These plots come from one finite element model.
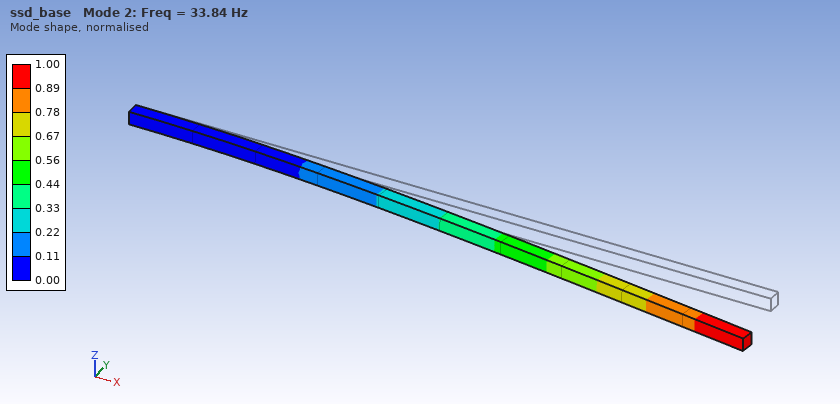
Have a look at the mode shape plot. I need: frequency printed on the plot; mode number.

33.84 Hz
2
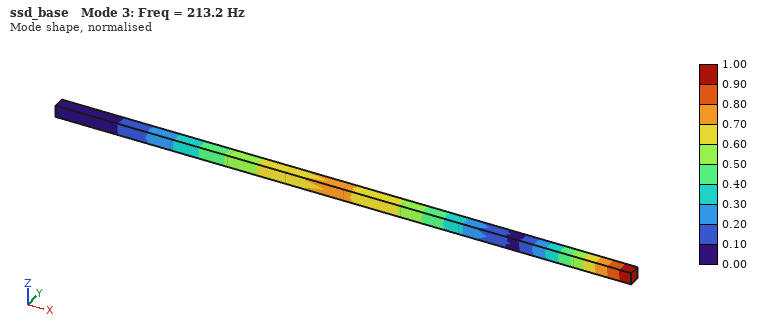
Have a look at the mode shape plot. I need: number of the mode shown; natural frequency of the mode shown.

3
213.2 Hz
